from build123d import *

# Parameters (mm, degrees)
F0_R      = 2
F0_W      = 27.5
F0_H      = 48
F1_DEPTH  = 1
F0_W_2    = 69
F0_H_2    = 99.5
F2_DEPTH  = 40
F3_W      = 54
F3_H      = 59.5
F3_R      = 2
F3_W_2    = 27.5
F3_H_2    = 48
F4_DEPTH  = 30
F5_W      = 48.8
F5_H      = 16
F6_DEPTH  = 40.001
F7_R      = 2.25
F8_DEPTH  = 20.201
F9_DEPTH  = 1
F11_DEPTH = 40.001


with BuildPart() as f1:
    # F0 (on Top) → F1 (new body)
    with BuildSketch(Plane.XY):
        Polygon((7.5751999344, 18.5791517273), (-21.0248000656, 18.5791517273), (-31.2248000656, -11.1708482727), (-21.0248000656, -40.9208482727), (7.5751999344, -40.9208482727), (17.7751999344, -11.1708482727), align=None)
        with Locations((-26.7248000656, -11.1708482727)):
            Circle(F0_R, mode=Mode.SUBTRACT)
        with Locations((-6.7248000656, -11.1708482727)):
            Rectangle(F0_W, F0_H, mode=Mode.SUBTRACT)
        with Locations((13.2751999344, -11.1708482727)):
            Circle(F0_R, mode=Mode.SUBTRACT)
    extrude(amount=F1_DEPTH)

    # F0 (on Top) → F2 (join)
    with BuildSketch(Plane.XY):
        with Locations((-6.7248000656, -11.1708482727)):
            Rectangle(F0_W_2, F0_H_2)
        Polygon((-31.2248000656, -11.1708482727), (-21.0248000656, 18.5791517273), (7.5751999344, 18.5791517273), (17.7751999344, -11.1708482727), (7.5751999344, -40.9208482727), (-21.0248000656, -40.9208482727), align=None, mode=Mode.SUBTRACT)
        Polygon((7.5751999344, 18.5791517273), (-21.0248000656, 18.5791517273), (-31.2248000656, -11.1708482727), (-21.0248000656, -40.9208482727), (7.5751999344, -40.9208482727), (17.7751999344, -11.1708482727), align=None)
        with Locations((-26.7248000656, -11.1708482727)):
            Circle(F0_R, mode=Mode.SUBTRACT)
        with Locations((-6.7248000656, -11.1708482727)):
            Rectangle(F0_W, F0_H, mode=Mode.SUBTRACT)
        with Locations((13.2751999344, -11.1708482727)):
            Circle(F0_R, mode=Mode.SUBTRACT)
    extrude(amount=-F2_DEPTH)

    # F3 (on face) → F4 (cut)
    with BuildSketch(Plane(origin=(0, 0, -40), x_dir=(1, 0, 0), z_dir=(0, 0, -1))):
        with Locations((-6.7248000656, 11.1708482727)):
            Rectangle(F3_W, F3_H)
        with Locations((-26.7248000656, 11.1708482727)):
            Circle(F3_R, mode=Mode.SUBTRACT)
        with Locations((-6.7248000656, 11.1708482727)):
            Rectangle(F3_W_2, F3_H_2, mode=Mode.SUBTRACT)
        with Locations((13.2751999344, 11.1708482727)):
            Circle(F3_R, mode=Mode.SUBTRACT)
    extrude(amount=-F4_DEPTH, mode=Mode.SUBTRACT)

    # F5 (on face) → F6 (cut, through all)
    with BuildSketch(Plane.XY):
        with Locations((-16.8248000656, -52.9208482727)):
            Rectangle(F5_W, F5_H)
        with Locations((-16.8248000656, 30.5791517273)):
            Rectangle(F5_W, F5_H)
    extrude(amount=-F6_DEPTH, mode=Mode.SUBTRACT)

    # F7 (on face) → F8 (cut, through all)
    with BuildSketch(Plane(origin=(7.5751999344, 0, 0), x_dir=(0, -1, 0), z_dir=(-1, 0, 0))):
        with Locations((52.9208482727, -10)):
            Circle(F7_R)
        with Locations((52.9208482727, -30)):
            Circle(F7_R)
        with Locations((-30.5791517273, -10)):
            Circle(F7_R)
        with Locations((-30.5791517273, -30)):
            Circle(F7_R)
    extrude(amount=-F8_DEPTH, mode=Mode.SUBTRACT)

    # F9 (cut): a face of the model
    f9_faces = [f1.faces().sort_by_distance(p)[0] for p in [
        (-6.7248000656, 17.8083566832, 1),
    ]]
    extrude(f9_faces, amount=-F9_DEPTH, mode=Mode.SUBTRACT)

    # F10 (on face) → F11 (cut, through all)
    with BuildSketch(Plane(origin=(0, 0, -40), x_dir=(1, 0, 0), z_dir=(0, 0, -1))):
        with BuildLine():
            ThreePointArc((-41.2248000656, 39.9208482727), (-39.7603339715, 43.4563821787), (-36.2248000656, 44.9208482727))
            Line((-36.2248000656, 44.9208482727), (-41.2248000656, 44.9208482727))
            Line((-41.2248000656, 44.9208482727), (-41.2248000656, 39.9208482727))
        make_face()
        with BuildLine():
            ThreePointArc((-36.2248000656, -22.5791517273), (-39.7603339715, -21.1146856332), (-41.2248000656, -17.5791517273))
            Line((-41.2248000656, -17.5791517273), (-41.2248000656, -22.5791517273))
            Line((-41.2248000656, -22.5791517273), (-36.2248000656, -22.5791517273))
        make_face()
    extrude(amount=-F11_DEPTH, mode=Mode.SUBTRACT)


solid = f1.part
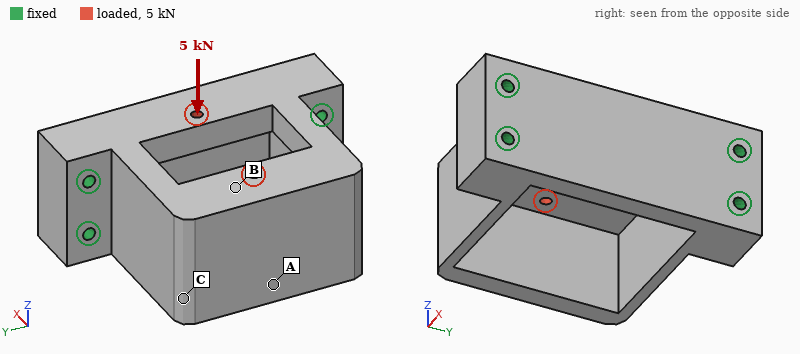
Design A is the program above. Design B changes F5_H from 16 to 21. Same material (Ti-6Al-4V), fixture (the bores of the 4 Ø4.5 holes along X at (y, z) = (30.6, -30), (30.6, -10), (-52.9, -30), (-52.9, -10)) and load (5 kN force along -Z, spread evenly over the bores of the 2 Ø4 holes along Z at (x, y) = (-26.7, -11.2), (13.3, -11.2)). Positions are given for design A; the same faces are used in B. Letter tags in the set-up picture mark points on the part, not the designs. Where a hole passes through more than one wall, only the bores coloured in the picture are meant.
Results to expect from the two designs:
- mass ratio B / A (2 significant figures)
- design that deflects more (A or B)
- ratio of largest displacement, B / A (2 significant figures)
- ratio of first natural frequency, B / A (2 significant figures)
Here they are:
0.91
B
1.5
0.74
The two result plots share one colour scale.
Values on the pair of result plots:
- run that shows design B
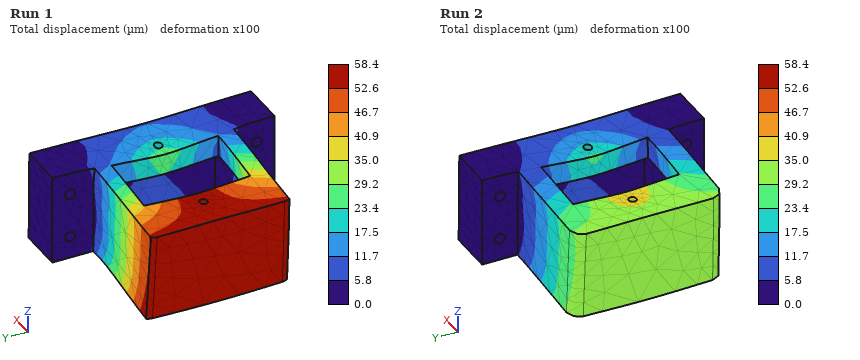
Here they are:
Run 1
